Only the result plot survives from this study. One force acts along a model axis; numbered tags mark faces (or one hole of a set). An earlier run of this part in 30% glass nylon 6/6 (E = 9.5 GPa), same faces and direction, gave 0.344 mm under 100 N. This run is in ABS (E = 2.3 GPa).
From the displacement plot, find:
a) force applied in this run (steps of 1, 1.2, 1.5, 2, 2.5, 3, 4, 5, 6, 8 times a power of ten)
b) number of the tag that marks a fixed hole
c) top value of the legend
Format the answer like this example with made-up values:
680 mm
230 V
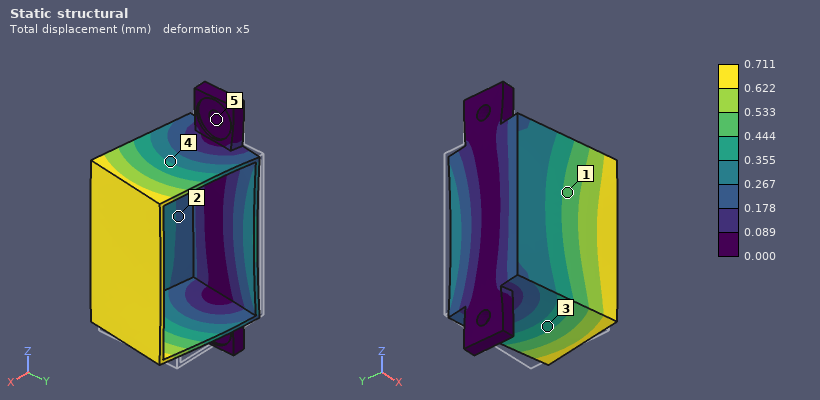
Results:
50 N
5
0.711 mm
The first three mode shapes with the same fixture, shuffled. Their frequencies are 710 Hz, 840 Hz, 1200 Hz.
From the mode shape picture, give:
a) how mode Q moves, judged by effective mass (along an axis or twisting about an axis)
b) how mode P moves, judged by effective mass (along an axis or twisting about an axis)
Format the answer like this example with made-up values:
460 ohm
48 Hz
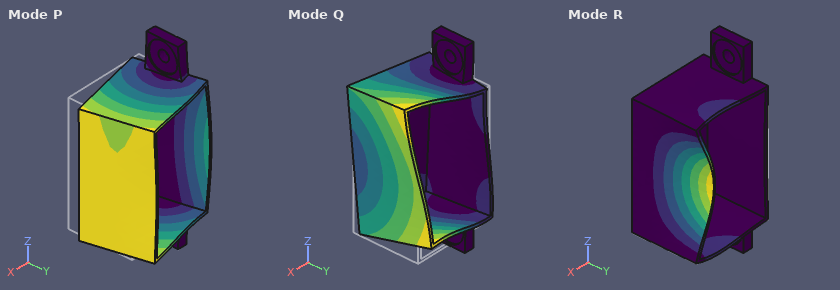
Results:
along Z
along Y
